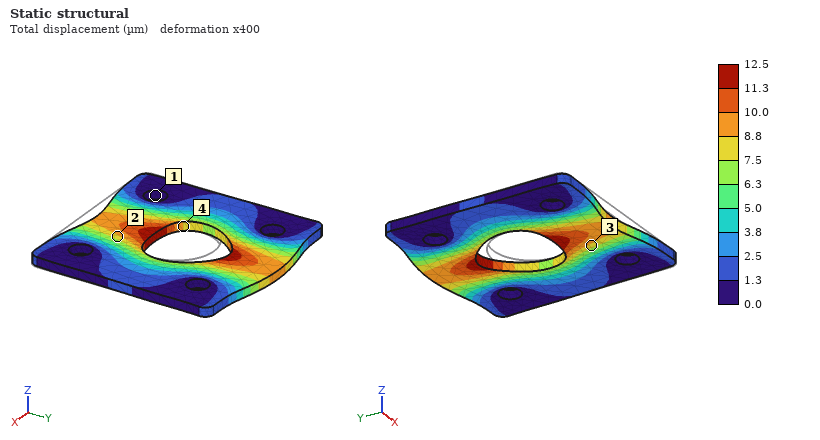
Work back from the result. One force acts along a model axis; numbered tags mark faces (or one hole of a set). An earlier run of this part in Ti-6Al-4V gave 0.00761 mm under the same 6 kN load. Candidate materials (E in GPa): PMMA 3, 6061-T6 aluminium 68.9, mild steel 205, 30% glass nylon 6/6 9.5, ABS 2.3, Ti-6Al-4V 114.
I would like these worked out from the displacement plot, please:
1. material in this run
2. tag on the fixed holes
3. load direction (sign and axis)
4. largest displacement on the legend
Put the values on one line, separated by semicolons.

6061-T6 aluminium; 1; +Y; 12.5 µm
